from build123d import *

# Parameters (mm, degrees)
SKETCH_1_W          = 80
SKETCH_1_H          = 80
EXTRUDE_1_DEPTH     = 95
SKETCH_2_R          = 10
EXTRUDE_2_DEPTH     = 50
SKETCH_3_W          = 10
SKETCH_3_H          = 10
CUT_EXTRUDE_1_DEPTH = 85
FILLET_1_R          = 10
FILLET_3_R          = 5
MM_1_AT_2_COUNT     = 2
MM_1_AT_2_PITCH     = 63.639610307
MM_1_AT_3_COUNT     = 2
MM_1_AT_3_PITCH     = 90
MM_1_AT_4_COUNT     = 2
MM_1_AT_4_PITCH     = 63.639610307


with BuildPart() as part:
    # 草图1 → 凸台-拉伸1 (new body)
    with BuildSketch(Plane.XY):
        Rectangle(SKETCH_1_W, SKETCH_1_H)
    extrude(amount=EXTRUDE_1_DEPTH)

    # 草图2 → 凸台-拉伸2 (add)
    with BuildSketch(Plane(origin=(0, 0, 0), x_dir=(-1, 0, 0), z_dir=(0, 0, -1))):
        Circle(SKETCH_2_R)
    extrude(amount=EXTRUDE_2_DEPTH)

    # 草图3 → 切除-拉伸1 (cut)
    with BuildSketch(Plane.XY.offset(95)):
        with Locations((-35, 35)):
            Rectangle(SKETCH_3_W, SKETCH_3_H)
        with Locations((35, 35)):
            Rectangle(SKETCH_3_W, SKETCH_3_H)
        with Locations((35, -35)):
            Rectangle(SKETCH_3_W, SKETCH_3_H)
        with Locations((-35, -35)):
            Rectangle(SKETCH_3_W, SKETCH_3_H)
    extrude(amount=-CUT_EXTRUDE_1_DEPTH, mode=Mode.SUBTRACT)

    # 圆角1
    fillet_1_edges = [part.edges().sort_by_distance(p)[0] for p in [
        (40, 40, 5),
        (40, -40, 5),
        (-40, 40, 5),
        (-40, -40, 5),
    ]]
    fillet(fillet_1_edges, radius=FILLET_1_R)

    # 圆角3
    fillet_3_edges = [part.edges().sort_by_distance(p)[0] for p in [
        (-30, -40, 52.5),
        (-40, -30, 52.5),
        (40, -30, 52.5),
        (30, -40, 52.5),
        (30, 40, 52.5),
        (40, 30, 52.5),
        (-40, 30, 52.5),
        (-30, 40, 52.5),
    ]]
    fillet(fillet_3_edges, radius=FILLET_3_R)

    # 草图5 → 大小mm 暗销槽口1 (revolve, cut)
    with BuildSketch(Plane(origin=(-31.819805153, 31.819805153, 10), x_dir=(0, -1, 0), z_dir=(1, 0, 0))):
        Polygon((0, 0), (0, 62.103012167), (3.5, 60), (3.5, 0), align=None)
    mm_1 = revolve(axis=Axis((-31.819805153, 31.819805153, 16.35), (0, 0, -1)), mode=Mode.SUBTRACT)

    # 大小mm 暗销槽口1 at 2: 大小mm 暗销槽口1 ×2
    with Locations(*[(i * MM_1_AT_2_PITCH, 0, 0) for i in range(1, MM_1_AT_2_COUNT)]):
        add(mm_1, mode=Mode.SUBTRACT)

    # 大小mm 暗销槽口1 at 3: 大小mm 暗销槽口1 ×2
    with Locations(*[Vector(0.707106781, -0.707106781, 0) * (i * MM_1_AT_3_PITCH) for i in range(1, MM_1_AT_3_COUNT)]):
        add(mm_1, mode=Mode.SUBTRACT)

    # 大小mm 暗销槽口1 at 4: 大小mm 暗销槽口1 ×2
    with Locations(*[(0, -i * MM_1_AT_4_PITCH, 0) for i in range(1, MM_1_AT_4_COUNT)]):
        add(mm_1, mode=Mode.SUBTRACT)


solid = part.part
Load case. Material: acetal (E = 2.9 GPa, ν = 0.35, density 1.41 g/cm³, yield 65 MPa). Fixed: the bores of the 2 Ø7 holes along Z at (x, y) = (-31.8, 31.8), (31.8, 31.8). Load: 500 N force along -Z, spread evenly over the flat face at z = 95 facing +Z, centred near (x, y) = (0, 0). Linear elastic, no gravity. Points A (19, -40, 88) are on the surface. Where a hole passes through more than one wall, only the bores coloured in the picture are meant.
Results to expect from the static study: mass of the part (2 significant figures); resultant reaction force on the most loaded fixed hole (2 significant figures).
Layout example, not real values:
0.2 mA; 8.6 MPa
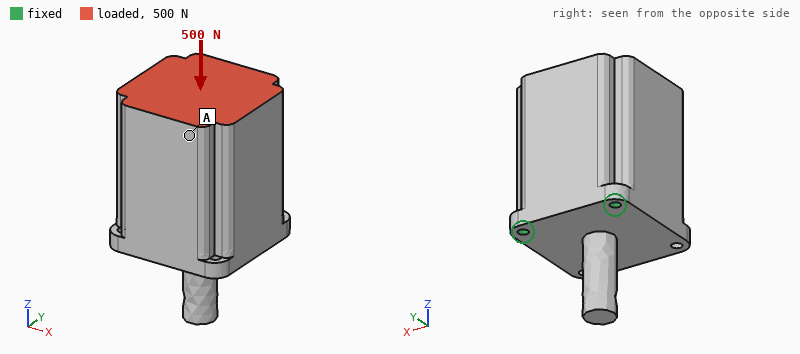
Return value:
820 g; 250 N
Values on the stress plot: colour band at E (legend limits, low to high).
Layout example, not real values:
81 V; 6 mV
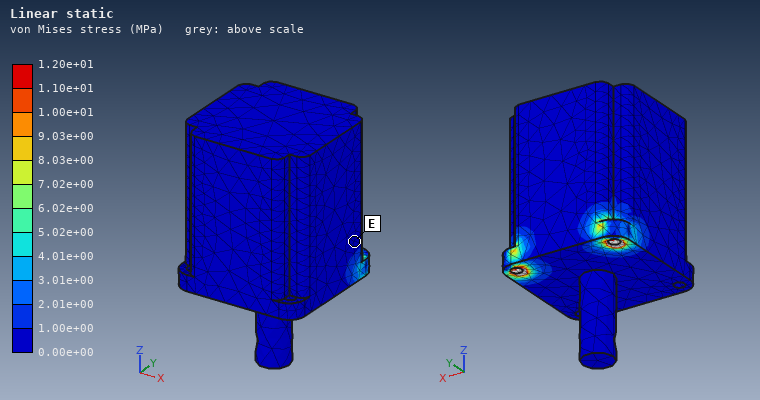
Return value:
0.00e+00 to 1.00e+00 MPa
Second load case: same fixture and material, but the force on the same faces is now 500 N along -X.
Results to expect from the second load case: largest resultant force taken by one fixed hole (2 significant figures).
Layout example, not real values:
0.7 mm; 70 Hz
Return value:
790 N
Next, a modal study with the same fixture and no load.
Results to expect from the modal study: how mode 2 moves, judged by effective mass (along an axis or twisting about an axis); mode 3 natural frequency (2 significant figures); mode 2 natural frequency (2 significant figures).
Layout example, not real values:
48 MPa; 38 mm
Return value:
along X; 1100 Hz; 710 Hz
